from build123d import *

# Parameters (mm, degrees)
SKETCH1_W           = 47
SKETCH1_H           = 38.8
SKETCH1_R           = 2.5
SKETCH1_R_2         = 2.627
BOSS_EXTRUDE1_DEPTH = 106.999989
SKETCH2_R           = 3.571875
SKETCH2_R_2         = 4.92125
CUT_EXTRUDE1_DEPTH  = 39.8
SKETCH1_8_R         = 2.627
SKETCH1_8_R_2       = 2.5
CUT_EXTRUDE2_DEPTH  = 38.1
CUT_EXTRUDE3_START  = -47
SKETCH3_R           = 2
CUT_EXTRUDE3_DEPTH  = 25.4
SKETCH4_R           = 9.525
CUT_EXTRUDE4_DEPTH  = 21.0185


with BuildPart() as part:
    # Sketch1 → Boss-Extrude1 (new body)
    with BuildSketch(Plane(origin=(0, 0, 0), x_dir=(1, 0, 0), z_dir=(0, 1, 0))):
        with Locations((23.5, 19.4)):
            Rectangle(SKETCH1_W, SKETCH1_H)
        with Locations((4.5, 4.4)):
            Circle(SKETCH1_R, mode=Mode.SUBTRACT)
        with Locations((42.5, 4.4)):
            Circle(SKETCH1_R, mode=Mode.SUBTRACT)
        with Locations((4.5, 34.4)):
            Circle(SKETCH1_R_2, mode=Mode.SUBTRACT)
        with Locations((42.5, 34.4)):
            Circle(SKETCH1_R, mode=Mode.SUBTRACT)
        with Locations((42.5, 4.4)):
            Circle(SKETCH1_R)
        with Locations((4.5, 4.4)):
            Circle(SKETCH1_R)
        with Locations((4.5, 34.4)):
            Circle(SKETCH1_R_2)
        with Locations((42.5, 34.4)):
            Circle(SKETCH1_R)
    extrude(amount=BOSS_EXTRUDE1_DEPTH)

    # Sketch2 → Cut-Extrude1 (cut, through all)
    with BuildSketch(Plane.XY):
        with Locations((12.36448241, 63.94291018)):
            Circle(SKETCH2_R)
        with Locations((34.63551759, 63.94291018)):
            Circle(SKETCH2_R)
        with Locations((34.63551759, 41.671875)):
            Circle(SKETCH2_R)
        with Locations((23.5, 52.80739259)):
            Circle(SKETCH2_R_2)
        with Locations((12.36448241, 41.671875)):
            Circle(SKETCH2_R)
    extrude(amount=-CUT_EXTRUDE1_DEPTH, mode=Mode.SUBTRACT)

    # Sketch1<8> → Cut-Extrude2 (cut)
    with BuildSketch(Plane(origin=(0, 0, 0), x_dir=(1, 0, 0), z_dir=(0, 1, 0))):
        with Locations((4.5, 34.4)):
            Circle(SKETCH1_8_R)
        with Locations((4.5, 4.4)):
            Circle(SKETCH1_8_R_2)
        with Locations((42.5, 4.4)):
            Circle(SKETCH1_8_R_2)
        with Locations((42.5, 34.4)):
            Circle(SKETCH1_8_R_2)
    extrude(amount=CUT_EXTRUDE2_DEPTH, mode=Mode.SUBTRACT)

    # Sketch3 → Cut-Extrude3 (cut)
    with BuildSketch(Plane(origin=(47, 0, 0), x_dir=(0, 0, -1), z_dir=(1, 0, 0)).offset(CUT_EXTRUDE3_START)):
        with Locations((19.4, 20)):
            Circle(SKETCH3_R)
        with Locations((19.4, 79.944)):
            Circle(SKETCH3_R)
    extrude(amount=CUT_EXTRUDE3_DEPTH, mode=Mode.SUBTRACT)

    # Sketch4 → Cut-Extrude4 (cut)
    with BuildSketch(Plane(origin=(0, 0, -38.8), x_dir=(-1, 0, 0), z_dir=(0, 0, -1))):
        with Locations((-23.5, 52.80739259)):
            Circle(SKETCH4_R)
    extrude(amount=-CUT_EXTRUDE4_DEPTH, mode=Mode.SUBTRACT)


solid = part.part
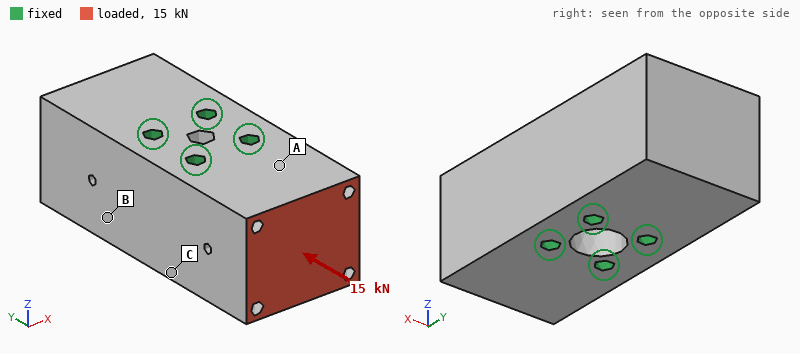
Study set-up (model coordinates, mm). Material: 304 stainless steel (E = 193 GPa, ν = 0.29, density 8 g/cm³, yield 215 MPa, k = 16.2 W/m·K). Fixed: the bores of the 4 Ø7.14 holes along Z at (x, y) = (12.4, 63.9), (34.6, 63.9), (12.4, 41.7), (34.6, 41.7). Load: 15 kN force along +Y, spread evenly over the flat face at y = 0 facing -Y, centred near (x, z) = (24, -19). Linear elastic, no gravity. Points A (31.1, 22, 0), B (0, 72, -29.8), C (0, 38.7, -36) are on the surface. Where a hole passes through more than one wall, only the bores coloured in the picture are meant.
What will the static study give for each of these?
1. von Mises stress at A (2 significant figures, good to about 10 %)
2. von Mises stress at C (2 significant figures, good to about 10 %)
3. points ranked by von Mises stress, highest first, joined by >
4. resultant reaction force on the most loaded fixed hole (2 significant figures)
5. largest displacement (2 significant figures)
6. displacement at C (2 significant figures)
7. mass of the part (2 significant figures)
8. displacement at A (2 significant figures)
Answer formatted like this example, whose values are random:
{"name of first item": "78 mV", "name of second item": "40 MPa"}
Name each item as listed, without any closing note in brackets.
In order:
{"von Mises stress at A": "8.6 MPa", "von Mises stress at C": "5.9 MPa", "points ranked by von Mises stress, highest first, joined by >": "A > C > B", "resultant reaction force on the most loaded fixed hole": "7.0 kN", "largest displacement": "2.0 µm", "displacement at C": "0.47 µm", "mass of the part": "1.4 kg", "displacement at A": "0.92 µm"}
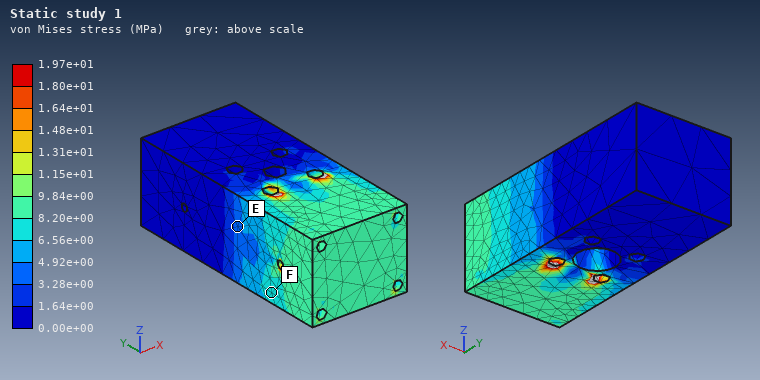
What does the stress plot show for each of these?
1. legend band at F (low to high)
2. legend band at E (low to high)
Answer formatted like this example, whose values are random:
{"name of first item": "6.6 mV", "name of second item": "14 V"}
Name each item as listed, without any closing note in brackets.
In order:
{"legend band at F": "6.56e+00 to 8.20e+00 MPa", "legend band at E": "3.28e+00 to 4.92e+00 MPa"}
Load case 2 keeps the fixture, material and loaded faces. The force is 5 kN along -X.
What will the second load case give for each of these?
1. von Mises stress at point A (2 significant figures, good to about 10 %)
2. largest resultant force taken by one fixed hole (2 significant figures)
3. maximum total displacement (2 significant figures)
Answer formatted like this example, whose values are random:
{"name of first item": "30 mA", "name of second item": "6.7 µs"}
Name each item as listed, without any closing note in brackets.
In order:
{"von Mises stress at point A": "7.7 MPa", "largest resultant force taken by one fixed hole": "6.5 kN", "maximum total displacement": "5.1 µm"}
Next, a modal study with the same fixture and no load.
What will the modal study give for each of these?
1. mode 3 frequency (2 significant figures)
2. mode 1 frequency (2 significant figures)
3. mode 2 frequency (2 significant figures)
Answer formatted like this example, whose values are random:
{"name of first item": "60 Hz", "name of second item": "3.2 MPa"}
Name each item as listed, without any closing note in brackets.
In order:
{"mode 3 frequency": "12 kHz", "mode 1 frequency": "11 kHz", "mode 2 frequency": "12 kHz"}
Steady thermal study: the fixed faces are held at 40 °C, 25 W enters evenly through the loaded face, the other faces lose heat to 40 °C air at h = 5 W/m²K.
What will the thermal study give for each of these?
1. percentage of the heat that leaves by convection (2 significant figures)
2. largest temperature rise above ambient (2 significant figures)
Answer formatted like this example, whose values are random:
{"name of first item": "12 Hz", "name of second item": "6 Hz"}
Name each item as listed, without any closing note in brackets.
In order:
{"percentage of the heat that leaves by convection": "3.6 %", "largest temperature rise above ambient": "36 K"}
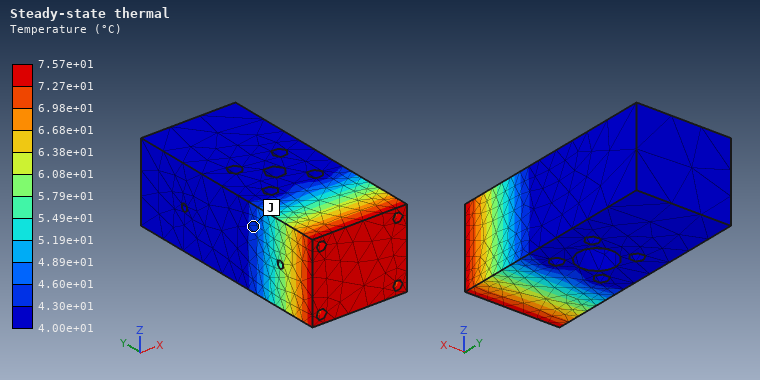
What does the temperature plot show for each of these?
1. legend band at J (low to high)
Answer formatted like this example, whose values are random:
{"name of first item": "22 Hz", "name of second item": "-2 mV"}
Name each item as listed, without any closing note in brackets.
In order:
{"legend band at J": "4.30e+01 to 4.60e+01 °C"}
